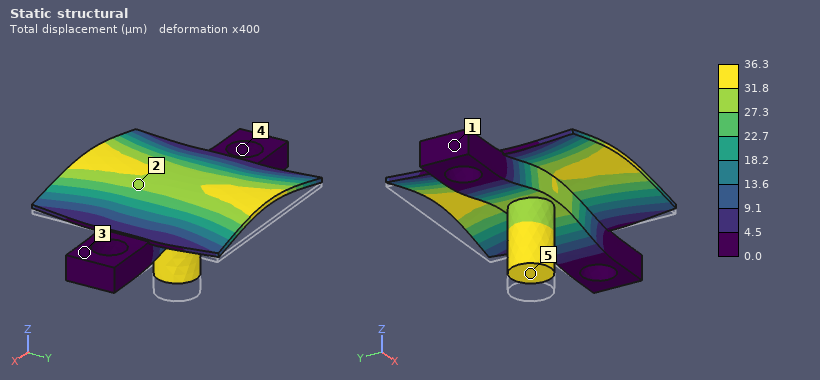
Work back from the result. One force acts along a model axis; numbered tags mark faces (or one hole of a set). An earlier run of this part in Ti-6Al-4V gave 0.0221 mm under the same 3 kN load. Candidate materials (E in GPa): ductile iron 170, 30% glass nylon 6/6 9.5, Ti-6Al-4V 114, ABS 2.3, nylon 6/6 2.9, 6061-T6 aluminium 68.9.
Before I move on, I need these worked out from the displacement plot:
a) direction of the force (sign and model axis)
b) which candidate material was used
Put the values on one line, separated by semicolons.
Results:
+Z; 6061-T6 aluminium
